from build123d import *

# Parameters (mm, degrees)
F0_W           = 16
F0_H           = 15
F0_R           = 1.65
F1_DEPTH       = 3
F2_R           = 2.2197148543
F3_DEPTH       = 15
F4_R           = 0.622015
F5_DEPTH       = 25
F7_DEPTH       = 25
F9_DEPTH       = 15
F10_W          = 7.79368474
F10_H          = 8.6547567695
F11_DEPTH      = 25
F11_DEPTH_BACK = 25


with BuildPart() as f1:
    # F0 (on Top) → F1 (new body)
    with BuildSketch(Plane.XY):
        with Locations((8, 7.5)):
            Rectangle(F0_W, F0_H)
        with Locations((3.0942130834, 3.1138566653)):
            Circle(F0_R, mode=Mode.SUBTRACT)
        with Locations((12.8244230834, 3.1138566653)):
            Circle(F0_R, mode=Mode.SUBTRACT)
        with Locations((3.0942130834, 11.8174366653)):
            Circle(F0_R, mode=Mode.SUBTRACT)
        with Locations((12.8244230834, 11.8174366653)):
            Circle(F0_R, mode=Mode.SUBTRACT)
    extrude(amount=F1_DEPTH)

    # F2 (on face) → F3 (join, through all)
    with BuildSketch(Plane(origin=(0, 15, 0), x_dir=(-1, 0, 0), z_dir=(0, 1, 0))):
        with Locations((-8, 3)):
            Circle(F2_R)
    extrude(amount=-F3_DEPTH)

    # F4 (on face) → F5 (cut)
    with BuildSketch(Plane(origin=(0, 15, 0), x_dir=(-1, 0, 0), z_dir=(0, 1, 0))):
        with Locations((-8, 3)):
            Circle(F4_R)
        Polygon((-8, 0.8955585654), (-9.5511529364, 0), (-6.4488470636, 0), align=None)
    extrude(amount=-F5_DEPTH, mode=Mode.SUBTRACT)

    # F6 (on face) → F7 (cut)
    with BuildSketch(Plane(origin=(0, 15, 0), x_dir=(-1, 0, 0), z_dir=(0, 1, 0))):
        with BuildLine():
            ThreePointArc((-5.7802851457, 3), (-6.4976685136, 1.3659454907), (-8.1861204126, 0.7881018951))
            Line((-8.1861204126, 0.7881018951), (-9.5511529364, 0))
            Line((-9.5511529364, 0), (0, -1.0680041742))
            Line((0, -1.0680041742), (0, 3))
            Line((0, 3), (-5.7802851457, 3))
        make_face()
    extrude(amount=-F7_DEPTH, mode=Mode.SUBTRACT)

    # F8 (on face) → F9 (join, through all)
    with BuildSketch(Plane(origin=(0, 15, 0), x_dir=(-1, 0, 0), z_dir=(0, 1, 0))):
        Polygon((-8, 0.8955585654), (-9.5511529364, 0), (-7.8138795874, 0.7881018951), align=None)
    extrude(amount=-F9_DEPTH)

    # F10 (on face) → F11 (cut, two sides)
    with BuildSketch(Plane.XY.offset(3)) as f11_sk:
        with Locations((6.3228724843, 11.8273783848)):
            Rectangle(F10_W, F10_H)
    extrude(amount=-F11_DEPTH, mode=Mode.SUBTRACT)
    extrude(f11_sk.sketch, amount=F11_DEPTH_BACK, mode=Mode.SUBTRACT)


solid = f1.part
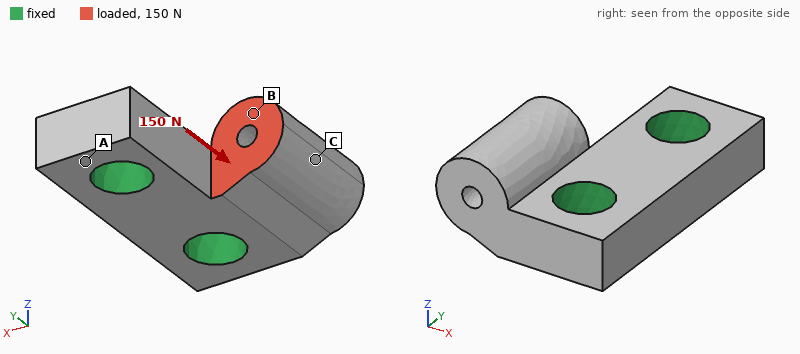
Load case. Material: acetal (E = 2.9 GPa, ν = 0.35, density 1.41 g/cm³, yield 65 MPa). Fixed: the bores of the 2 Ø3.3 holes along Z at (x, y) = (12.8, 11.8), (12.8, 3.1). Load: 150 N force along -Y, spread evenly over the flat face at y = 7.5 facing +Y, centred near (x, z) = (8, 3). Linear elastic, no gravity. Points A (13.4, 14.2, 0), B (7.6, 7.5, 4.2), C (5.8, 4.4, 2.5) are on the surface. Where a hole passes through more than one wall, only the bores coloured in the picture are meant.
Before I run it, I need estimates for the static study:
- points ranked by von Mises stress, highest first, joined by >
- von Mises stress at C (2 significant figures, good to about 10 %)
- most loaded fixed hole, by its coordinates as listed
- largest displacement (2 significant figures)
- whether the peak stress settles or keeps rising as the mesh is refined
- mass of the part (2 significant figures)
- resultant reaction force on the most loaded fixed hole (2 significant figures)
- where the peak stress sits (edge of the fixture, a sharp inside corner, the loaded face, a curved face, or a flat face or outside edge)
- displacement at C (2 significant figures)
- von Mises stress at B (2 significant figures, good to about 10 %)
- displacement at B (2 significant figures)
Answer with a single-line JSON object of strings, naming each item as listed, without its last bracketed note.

{"points ranked by von Mises stress, highest first, joined by >": "B > C > A", "von Mises stress at C": "6.5 MPa", "most loaded fixed hole, by its coordinates as listed": "(12.8, 3.1)", "largest displacement": "71 µm", "whether the peak stress settles or keeps rising as the mesh is refined": "keeps rising", "mass of the part": "0.47 g", "resultant reaction force on the most loaded fixed hole": "120 N", "where the peak stress sits": "a sharp inside corner", "displacement at C": "49 µm", "von Mises stress at B": "8.6 MPa", "displacement at B": "61 µm"}
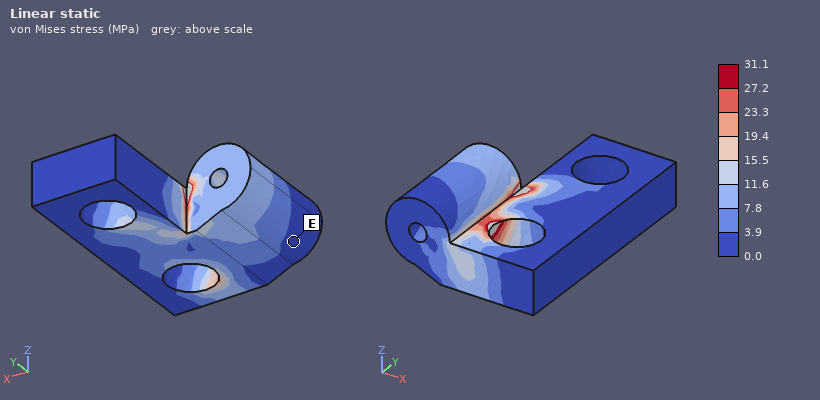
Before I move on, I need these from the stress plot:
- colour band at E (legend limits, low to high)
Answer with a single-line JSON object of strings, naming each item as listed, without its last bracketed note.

{"colour band at E": "0.0 to 3.9 MPa"}
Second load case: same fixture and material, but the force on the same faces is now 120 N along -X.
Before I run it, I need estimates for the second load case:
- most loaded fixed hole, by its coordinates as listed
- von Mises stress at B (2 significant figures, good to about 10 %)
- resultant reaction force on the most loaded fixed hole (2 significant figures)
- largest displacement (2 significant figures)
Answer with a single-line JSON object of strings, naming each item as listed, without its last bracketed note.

{"most loaded fixed hole, by its coordinates as listed": "(12.8, 3.1)", "von Mises stress at B": "23 MPa", "resultant reaction force on the most loaded fixed hole": "77 N", "largest displacement": "0.11 mm"}
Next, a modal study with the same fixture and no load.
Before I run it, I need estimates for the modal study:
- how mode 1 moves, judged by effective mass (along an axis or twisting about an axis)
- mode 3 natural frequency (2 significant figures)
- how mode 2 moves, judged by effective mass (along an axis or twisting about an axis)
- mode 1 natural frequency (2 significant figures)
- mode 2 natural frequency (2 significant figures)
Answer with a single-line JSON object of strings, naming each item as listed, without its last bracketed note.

{"how mode 1 moves, judged by effective mass": "along Z", "mode 3 natural frequency": "26 kHz", "how mode 2 moves, judged by effective mass": "along Y", "mode 1 natural frequency": "14 kHz", "mode 2 natural frequency": "21 kHz"}
